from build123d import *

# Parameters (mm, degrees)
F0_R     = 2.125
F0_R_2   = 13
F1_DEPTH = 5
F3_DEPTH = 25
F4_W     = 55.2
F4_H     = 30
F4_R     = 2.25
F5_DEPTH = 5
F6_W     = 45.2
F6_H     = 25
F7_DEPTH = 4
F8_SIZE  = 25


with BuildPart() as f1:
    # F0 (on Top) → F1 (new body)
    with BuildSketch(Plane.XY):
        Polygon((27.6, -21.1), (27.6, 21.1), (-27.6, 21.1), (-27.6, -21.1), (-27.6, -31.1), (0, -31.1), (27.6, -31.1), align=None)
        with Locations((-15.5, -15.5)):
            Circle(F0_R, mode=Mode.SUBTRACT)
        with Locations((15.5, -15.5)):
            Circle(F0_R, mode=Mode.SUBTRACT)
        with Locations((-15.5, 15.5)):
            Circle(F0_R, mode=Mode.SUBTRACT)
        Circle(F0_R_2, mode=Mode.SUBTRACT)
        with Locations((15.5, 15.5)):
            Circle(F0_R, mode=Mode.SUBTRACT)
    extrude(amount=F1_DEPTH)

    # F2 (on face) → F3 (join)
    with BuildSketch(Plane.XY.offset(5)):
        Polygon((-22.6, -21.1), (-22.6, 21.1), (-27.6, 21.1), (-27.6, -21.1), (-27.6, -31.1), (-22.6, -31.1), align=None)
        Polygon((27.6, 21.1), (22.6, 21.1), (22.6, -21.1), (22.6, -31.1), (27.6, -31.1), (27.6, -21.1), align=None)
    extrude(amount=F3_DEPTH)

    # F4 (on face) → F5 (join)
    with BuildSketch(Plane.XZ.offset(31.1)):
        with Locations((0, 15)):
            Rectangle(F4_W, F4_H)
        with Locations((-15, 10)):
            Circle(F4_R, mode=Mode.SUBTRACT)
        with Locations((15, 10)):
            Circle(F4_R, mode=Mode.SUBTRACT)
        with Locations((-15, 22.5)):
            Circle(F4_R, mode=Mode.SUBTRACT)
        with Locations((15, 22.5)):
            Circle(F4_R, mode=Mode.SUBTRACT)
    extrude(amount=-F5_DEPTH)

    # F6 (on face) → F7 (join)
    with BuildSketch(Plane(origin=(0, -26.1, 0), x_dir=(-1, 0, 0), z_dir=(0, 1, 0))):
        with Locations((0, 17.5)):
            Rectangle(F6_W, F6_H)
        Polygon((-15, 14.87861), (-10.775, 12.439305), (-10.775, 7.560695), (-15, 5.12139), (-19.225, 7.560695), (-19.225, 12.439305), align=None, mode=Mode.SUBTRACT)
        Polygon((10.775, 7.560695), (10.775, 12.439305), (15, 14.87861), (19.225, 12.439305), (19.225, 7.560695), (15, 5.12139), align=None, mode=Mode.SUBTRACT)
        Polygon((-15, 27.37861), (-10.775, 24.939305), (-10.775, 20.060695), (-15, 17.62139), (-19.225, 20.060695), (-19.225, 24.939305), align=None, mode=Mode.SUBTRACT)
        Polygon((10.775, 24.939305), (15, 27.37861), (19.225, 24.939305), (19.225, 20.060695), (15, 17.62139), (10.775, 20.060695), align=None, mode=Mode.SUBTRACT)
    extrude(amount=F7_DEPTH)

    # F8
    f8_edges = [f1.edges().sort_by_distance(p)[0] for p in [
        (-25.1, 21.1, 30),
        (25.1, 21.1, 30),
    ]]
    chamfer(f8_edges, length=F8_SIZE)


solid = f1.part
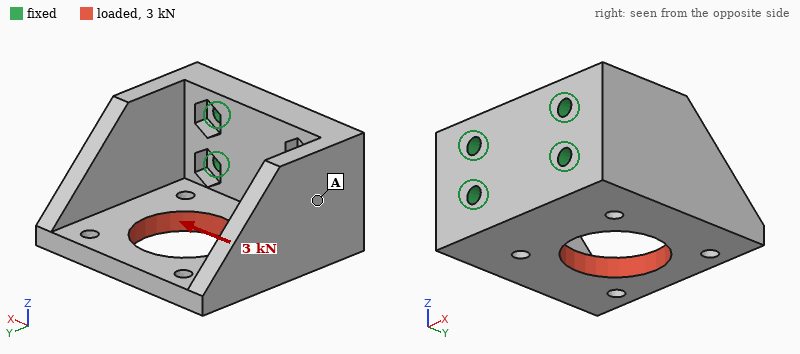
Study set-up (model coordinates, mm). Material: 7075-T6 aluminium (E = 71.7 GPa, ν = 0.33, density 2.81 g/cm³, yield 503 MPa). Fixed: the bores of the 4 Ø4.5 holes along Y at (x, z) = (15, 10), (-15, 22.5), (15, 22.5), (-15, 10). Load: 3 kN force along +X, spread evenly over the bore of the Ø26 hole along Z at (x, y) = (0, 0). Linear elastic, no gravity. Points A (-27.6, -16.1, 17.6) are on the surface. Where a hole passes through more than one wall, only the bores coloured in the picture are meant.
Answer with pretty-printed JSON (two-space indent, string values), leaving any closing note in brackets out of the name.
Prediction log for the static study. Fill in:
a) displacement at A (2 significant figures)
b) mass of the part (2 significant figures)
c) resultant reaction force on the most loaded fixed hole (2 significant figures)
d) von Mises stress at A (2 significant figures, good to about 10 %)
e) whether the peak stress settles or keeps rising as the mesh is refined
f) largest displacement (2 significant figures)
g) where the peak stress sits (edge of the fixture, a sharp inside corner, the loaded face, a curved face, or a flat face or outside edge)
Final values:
{
  "displacement at A": "22 µm",
  "mass of the part": "85 g",
  "resultant reaction force on the most loaded fixed hole": "2.7 kN",
  "von Mises stress at A": "13 MPa",
  "whether the peak stress settles or keeps rising as the mesh is refined": "keeps rising",
  "largest displacement": "96 µm",
  "where the peak stress sits": "edge of the fixture"
}
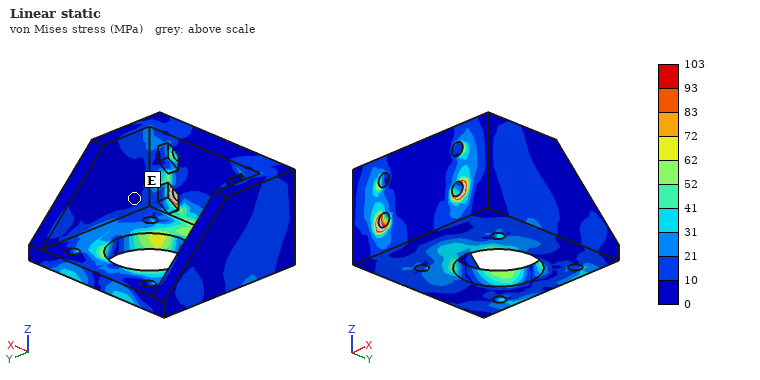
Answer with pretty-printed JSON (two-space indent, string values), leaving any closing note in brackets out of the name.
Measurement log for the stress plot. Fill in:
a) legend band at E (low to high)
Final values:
{
  "legend band at E": "0 to 10 MPa"
}
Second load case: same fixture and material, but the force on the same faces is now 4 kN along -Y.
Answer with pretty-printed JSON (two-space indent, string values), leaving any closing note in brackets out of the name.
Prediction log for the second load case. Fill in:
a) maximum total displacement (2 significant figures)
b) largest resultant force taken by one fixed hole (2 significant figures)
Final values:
{
  "maximum total displacement": "56 µm",
  "largest resultant force taken by one fixed hole": "2.6 kN"
}
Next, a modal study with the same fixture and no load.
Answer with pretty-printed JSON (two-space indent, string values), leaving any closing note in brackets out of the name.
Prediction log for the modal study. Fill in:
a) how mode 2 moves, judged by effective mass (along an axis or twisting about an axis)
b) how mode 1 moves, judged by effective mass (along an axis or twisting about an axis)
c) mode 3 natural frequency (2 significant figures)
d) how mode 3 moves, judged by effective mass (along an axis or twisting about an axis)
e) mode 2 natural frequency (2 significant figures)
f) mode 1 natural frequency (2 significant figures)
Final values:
{
  "how mode 2 moves, judged by effective mass": "along X",
  "how mode 1 moves, judged by effective mass": "along Z",
  "mode 3 natural frequency": "7200 Hz",
  "how mode 3 moves, judged by effective mass": "along X",
  "mode 2 natural frequency": "4700 Hz",
  "mode 1 natural frequency": "4300 Hz"
}
